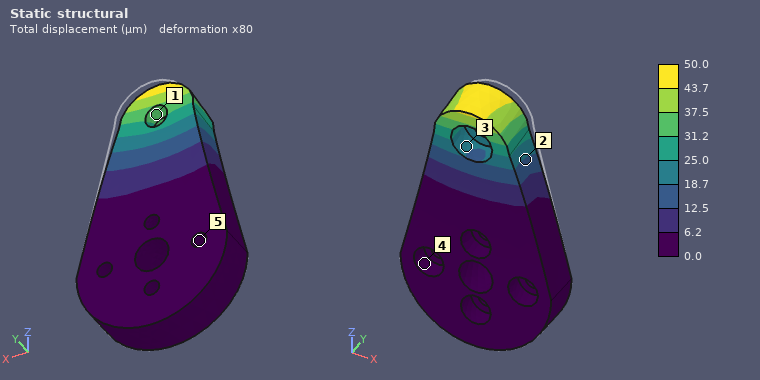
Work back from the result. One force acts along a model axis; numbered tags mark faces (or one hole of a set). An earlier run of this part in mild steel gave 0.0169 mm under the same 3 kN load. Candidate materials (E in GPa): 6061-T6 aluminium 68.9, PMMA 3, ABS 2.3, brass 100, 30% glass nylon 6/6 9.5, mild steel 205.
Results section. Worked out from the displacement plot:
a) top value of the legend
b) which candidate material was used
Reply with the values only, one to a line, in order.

50.0 µm
6061-T6 aluminium
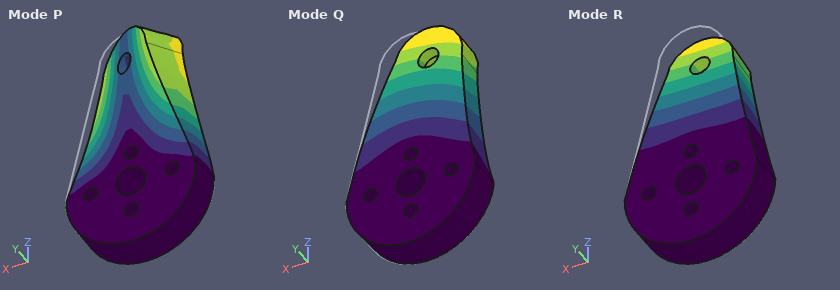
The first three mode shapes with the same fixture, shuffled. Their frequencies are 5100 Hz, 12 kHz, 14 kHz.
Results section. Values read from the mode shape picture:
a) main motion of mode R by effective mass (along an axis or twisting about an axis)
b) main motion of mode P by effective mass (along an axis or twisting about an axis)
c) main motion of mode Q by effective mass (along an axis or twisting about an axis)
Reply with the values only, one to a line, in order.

along Y
twisting about Z
along X
